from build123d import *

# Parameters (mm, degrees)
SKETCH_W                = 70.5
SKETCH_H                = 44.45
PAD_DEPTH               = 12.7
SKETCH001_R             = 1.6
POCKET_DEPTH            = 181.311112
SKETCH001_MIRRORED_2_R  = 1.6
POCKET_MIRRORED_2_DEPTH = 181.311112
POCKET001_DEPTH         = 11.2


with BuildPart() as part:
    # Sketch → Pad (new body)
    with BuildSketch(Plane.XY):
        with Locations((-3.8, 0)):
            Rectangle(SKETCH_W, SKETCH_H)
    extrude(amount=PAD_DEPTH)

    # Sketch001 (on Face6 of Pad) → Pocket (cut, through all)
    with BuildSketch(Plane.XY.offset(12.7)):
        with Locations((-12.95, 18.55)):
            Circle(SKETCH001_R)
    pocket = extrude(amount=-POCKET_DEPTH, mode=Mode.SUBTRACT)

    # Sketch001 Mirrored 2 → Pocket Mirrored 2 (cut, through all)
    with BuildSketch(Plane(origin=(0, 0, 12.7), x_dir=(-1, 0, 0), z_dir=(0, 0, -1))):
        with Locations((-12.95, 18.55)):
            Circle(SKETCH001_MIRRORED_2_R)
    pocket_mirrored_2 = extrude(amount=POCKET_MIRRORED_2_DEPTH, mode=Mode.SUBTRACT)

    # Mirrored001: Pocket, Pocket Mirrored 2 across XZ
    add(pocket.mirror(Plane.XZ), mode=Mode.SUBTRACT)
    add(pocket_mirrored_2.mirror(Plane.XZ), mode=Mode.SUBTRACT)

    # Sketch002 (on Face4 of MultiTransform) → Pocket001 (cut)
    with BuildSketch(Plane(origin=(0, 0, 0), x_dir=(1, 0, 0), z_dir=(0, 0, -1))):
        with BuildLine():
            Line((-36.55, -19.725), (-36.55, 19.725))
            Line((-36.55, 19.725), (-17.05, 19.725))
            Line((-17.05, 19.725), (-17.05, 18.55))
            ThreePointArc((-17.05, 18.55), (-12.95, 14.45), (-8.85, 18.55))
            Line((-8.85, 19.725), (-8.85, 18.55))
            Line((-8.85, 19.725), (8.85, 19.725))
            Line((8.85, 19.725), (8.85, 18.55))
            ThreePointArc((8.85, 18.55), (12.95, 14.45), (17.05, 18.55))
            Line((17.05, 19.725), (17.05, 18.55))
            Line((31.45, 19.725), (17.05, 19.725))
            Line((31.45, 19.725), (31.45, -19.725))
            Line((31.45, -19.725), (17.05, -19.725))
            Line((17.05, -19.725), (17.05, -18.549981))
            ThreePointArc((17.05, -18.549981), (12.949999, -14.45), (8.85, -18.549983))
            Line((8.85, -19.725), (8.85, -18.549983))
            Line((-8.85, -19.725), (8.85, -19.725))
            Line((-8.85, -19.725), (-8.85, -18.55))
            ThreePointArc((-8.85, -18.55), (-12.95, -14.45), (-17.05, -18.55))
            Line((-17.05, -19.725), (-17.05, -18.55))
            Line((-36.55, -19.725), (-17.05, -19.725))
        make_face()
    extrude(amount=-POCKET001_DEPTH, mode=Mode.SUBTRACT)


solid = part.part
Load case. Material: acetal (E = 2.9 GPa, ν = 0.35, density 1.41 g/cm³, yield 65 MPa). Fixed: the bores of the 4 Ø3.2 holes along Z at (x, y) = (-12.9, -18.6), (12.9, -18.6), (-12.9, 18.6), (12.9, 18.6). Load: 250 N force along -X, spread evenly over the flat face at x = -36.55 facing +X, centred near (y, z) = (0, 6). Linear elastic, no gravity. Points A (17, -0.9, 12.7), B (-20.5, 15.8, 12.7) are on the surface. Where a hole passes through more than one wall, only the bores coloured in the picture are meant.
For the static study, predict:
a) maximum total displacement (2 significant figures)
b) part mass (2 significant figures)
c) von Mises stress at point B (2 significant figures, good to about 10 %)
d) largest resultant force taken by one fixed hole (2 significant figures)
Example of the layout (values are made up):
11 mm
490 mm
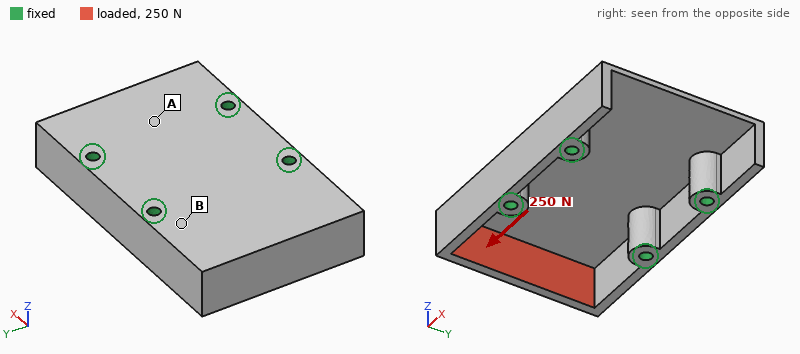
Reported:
0.83 mm
15 g
6.1 MPa
110 N
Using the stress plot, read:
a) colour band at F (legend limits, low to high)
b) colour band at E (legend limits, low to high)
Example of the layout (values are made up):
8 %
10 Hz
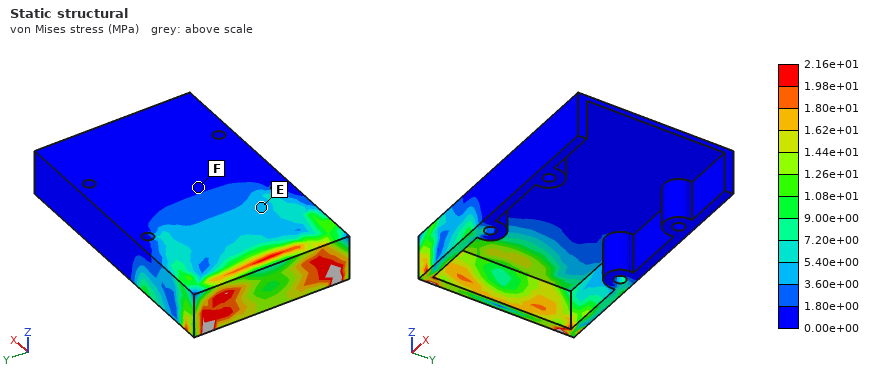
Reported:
0.00e+00 to 1.80e+00 MPa
3.60e+00 to 5.40e+00 MPa
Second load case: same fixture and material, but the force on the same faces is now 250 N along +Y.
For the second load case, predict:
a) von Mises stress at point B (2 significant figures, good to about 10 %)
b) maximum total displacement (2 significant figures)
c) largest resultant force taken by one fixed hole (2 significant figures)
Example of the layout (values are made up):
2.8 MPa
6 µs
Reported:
8.4 MPa
0.33 mm
190 N
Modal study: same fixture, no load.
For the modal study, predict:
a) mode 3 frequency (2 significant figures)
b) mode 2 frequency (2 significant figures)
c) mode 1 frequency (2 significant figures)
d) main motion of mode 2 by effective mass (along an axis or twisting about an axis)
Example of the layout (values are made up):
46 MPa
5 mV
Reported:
2100 Hz
2000 Hz
1600 Hz
along Z
